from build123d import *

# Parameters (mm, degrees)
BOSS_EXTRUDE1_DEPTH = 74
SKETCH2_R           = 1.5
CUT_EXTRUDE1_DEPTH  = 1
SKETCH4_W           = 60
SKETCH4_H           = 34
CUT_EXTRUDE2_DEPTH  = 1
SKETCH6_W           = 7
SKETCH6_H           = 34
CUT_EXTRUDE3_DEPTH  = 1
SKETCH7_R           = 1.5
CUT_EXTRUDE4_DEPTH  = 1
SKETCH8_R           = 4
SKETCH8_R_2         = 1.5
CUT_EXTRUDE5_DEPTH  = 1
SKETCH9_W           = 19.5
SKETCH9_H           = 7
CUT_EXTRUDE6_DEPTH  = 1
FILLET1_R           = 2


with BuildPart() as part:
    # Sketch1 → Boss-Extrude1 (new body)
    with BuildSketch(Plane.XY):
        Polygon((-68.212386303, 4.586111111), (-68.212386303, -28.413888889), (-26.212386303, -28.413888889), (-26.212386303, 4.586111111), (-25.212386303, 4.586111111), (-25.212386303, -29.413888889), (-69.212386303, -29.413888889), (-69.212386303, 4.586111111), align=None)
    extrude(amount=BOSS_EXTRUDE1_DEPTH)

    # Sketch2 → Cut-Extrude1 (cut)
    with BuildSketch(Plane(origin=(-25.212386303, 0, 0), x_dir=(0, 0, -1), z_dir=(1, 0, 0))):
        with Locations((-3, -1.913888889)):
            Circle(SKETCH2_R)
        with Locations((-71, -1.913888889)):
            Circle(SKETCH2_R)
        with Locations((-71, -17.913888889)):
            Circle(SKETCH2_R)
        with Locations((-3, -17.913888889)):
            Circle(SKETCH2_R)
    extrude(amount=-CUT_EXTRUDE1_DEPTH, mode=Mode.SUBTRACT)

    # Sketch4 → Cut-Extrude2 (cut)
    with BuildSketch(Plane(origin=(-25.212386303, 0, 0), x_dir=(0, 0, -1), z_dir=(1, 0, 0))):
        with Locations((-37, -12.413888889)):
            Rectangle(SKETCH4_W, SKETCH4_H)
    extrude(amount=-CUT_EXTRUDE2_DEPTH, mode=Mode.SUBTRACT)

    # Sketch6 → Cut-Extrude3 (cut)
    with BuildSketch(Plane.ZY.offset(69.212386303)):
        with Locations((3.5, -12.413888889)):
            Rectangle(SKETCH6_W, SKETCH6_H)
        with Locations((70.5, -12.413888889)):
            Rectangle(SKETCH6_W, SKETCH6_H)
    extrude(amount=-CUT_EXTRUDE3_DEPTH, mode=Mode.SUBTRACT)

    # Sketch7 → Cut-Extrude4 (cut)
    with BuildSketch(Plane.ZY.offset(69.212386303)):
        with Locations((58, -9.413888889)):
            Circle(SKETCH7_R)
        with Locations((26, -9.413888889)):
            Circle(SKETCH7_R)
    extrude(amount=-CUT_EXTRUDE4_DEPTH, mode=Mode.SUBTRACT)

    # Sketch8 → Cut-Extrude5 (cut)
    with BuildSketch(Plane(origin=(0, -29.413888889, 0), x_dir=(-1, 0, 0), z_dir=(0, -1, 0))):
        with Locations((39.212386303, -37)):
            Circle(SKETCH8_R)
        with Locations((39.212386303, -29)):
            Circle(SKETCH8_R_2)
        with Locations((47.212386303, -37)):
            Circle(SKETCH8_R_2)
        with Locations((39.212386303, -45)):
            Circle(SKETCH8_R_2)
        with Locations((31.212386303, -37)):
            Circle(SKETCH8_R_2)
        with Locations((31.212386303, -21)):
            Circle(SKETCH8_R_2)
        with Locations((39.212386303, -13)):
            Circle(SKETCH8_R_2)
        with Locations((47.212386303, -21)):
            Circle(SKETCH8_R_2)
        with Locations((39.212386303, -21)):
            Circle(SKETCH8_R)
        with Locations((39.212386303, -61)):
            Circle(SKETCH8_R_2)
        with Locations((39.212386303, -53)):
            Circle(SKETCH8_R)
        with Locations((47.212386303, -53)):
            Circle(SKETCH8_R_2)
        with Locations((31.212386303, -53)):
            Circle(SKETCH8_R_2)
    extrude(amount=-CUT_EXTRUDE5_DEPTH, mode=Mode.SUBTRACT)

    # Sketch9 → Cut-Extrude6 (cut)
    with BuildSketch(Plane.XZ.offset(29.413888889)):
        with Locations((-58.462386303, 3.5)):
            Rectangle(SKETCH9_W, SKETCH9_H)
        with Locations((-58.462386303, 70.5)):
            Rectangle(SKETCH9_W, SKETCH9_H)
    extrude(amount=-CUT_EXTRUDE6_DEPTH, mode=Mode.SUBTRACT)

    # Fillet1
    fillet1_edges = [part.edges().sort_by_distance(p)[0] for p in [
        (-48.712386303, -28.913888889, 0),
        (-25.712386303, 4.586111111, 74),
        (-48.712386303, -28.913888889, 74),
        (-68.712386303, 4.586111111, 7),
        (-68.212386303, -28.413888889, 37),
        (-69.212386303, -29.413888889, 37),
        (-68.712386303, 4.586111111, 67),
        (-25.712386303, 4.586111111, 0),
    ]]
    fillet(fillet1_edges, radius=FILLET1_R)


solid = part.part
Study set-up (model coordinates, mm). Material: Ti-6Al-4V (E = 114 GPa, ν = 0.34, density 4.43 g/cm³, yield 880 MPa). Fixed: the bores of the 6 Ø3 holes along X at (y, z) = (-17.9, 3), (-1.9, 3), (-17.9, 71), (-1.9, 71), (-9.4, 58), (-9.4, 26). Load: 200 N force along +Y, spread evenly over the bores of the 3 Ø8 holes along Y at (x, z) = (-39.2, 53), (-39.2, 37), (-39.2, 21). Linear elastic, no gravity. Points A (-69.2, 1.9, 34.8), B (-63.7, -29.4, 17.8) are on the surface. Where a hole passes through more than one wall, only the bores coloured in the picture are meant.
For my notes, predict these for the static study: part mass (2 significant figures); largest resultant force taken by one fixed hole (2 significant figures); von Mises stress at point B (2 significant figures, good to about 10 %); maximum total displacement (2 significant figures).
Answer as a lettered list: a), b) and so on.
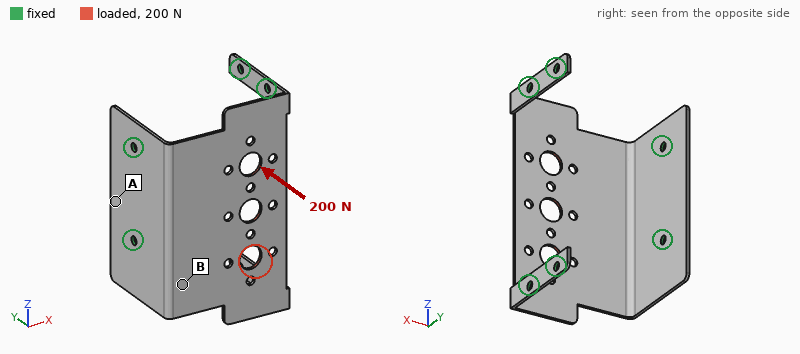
a) 23 g
b) 95 N
c) 80 MPa
d) 0.96 mm
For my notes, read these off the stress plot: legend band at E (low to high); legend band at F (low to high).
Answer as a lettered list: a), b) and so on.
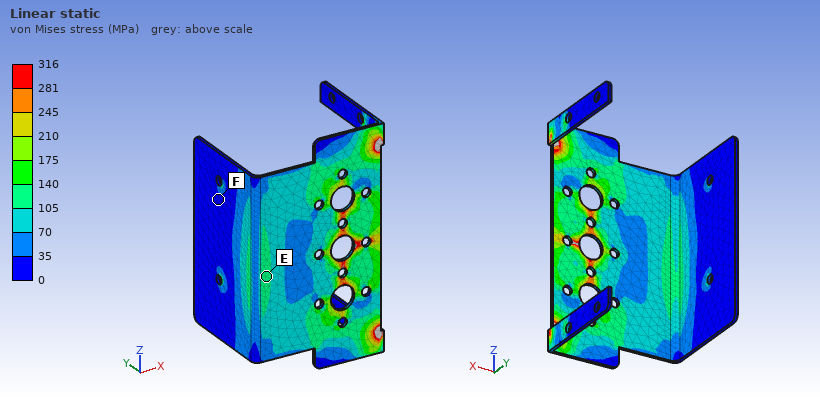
a) 105 to 140 MPa
b) 0 to 35 MPa
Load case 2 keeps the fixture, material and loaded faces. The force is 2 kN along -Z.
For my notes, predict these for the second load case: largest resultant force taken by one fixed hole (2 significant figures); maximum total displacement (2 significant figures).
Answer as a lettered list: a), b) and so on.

a) 770 N
b) 0.20 mm
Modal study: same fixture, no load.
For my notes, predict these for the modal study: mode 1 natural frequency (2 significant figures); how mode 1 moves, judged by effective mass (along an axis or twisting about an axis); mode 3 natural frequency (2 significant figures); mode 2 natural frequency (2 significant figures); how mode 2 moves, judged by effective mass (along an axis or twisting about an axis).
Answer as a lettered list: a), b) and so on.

a) 1300 Hz
b) along Y
c) 2200 Hz
d) 1600 Hz
e) along X
